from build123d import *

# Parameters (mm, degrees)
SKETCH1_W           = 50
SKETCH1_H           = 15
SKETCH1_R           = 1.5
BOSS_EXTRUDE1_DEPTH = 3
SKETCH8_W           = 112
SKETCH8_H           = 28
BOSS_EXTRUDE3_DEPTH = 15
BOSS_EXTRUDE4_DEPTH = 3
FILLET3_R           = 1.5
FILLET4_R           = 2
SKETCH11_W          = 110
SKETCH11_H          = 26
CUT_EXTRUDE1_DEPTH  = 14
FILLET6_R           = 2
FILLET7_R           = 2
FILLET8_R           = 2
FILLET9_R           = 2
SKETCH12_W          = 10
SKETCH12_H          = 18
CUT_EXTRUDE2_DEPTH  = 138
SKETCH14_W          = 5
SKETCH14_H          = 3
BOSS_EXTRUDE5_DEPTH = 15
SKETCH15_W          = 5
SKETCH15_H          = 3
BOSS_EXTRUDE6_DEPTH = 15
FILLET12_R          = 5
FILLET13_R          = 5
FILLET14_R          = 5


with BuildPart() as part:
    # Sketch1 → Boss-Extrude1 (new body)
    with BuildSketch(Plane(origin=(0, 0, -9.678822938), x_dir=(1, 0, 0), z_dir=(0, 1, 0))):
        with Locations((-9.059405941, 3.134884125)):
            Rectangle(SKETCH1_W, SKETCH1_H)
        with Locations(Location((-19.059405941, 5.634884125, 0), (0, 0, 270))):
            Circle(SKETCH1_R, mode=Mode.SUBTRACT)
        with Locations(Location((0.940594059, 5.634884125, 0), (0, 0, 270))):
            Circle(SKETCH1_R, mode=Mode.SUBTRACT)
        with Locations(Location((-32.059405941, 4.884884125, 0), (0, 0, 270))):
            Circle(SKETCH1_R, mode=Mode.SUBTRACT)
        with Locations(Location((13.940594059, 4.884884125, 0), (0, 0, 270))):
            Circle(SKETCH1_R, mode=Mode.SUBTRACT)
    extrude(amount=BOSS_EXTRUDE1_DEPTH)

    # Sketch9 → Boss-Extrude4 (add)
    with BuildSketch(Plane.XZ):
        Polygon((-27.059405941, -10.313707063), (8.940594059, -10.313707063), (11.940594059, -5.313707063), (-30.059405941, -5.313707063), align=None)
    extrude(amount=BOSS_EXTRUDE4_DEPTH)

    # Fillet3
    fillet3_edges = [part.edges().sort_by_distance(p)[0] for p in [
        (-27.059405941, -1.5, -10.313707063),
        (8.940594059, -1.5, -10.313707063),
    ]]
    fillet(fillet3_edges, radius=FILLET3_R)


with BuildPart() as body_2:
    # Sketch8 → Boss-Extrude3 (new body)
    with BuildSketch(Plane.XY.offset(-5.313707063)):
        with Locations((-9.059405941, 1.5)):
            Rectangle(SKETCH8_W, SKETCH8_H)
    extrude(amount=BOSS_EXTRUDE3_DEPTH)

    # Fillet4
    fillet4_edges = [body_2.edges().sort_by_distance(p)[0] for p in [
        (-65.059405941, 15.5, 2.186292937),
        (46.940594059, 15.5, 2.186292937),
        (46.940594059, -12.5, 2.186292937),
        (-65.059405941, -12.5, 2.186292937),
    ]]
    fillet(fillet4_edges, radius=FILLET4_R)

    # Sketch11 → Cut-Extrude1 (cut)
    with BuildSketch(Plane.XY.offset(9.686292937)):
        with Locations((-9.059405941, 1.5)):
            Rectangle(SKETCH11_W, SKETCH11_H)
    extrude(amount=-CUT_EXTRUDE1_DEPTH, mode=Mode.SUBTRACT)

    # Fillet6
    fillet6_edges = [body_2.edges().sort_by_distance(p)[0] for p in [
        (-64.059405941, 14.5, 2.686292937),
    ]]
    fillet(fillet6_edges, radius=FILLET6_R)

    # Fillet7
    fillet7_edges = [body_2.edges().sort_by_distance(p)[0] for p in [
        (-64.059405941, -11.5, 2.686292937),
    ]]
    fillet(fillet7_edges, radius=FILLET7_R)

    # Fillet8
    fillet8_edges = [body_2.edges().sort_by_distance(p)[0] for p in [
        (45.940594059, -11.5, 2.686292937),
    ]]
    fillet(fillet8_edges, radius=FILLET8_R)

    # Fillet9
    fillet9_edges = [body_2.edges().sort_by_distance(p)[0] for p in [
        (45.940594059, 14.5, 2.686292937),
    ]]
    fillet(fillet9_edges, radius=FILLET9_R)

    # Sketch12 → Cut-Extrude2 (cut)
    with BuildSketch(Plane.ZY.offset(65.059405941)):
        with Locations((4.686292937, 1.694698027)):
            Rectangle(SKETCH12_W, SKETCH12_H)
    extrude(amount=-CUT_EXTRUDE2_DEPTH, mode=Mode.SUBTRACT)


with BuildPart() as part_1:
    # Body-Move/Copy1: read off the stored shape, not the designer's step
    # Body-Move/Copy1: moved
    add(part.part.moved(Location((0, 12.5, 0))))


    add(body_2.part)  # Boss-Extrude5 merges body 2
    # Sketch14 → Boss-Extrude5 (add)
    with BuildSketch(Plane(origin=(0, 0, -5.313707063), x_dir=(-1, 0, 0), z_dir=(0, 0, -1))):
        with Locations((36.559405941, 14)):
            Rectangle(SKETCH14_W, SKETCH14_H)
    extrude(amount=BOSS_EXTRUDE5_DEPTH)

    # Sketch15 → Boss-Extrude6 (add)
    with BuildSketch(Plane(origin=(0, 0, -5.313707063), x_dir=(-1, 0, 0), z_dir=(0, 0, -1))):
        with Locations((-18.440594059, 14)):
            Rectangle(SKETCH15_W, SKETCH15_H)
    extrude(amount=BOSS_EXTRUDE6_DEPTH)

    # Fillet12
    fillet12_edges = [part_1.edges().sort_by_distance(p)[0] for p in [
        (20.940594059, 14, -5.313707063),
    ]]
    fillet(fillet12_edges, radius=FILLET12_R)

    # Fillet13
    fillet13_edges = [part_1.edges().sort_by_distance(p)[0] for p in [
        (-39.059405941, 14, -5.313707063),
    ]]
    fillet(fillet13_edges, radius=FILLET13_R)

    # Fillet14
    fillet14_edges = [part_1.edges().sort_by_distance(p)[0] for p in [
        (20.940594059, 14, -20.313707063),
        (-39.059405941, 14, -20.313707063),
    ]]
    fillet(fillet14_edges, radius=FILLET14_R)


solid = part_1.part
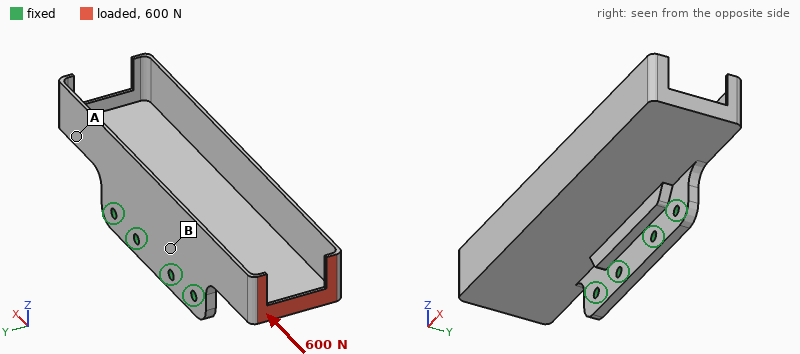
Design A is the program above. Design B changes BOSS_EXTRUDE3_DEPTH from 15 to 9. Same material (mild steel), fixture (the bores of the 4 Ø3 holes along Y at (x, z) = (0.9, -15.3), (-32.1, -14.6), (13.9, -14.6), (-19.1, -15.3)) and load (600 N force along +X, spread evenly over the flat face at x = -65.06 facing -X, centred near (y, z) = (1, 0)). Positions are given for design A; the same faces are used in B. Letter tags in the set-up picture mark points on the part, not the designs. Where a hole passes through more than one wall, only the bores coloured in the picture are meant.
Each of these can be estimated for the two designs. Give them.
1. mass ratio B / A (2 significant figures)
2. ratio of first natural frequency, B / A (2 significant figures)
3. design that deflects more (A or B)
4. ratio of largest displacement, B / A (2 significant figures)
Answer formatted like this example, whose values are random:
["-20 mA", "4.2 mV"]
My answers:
["0.85", "1.2", "A", "0.70"]
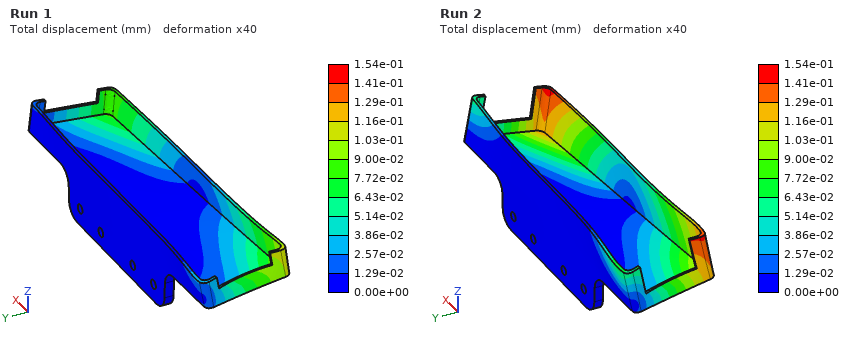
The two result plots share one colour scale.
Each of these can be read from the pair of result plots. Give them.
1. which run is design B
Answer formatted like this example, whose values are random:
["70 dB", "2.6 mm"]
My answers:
["Run 1"]
